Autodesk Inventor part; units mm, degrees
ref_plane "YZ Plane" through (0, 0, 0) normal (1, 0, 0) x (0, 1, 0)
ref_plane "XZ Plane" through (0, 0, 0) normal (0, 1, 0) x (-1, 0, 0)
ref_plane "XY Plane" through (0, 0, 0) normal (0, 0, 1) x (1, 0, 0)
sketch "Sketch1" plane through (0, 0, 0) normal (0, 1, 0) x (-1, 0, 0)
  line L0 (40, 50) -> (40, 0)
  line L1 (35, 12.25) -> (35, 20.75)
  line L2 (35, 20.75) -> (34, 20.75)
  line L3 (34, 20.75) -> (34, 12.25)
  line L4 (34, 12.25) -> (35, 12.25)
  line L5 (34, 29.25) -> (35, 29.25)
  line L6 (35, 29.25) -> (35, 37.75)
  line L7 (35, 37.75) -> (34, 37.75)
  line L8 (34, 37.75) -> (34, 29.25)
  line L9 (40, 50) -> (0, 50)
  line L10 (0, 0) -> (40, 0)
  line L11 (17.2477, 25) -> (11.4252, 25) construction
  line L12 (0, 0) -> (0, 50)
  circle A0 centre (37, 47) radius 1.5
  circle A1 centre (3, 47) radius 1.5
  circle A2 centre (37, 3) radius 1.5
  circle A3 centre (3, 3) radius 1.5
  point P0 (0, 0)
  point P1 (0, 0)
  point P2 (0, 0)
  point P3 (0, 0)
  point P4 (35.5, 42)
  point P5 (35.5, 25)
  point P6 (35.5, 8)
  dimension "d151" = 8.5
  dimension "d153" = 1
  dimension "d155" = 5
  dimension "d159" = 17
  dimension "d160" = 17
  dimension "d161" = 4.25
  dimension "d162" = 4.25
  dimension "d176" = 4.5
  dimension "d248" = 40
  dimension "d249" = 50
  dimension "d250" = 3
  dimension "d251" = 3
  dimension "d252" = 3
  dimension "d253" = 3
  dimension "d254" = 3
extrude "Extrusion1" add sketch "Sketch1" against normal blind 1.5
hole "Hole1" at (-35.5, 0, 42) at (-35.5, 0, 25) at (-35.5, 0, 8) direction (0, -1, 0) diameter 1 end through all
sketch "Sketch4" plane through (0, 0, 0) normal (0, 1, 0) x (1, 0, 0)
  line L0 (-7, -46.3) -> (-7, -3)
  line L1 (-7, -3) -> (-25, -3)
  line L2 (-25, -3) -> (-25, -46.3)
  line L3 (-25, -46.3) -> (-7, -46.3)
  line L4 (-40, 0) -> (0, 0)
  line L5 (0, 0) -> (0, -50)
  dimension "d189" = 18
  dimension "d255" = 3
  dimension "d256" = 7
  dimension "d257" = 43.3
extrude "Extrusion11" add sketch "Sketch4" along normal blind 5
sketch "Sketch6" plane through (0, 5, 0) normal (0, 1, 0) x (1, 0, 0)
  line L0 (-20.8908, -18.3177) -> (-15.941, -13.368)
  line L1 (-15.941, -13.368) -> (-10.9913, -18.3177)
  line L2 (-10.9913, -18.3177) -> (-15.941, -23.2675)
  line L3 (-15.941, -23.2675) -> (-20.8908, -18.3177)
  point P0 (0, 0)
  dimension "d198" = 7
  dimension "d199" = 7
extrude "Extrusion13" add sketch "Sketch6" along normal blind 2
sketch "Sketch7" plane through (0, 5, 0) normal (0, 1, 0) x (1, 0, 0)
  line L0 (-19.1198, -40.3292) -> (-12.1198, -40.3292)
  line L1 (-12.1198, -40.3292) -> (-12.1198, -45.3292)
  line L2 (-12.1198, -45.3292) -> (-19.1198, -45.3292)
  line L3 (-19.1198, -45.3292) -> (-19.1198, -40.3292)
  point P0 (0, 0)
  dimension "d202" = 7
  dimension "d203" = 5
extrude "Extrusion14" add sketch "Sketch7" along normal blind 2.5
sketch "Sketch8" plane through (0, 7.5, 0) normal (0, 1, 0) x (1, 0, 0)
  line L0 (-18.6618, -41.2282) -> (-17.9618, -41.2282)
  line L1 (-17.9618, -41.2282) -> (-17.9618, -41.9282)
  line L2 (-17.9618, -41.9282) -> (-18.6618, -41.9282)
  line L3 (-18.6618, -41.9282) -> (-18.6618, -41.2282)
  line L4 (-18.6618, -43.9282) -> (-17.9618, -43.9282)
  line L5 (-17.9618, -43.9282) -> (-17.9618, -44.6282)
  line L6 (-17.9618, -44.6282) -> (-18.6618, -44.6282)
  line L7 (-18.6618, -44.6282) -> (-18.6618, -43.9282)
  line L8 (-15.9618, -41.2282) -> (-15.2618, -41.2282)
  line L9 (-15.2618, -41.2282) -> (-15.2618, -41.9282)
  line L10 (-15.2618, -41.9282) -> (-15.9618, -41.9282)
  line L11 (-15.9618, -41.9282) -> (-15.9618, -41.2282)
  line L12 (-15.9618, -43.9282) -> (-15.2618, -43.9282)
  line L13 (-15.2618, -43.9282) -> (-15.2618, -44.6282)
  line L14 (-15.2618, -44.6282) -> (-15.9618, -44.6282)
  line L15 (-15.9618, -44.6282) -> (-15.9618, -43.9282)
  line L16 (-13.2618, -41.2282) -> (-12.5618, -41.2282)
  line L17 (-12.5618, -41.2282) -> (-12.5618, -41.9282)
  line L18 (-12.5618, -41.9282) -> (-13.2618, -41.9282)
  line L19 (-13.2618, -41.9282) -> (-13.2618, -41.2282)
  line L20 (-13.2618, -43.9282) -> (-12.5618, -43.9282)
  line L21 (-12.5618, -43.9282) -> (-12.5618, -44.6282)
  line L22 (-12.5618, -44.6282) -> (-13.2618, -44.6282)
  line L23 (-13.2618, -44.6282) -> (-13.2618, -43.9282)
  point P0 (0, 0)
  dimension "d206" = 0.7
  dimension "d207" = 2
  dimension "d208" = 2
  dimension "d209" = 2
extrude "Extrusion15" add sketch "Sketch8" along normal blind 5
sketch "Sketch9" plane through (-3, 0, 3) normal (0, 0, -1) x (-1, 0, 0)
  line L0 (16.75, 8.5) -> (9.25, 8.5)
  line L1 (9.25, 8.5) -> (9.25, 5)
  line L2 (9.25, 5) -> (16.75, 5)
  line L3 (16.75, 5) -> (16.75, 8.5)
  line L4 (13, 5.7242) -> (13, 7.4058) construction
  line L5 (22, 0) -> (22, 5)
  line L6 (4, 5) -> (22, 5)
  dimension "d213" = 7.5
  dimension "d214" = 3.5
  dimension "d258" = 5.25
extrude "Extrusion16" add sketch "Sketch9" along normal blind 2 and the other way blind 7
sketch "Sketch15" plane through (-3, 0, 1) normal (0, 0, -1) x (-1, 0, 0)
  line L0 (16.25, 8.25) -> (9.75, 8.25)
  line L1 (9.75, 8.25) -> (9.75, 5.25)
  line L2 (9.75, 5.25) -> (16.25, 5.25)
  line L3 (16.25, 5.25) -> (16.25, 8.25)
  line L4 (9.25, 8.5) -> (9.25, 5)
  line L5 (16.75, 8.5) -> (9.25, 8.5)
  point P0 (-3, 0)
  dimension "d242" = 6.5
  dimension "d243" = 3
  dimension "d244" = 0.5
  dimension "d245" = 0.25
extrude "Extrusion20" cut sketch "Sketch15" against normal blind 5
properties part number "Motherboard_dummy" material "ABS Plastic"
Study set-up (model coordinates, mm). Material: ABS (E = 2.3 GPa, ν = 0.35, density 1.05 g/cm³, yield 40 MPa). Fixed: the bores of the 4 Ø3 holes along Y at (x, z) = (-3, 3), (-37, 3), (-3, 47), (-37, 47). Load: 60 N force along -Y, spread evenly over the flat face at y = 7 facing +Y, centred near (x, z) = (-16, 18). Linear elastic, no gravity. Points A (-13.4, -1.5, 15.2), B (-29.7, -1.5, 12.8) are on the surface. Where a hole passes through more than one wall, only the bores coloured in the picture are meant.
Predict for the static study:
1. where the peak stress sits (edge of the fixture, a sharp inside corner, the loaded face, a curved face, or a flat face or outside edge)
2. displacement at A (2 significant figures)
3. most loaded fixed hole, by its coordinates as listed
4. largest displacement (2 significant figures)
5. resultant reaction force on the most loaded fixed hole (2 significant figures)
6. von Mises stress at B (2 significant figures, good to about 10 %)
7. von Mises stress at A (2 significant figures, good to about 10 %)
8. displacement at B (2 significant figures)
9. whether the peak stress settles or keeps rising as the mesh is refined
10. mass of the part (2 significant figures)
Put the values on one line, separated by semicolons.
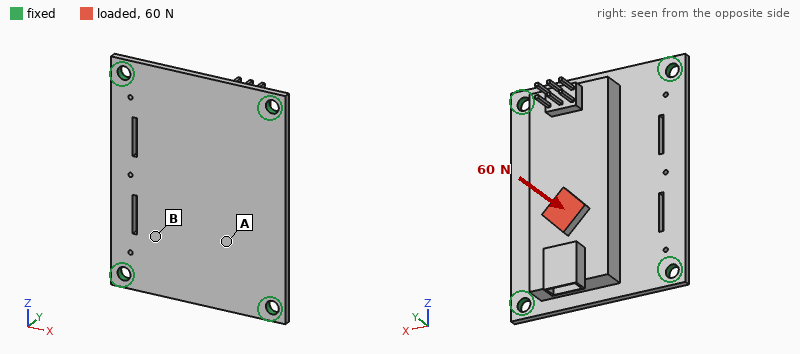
edge of the fixture; 0.14 mm; (-3, 3); 0.23 mm; 36 N; 4.3 MPa; 2.0 MPa; 0.20 mm; keeps rising; 7.5 g
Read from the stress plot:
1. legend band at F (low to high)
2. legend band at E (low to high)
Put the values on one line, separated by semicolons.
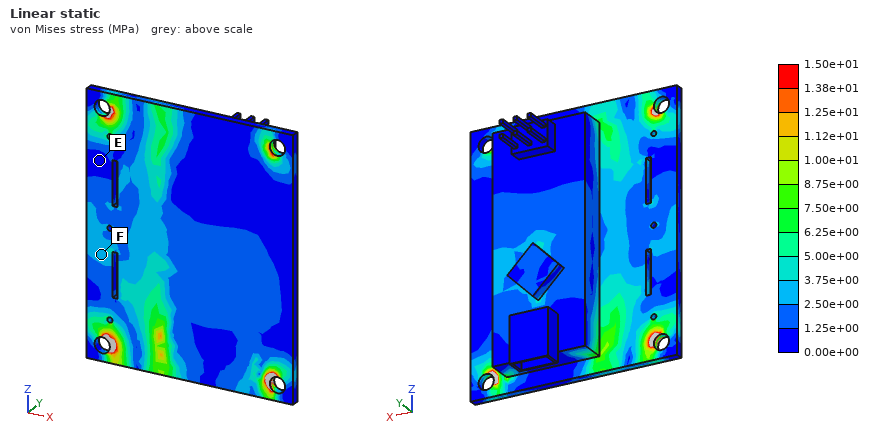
2.50e+00 to 3.75e+00 MPa; 0.00e+00 to 1.25e+00 MPa
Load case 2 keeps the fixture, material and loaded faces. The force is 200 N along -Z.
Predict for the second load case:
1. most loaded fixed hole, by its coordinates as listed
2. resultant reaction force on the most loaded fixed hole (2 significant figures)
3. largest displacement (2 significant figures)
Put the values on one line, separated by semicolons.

(-3, 47); 94 N; 0.14 mm
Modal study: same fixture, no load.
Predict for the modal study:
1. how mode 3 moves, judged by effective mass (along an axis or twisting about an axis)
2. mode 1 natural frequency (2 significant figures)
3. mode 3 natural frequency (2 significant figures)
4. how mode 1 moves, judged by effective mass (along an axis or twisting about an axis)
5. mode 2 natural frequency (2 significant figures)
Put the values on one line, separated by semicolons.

twisting about X; 1200 Hz; 2600 Hz; along Y; 2400 Hz
